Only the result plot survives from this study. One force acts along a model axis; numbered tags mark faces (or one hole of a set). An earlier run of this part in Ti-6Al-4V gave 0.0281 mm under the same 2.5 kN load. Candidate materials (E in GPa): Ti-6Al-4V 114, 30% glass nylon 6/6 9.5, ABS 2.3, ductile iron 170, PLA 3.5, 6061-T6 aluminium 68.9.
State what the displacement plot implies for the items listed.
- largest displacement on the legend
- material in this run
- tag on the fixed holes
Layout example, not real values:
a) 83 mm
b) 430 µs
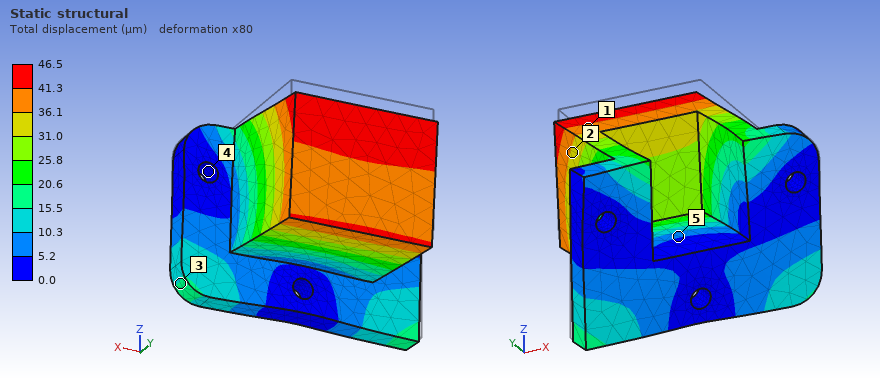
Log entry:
a) 46.5 µm
b) 6061-T6 aluminium
c) 4
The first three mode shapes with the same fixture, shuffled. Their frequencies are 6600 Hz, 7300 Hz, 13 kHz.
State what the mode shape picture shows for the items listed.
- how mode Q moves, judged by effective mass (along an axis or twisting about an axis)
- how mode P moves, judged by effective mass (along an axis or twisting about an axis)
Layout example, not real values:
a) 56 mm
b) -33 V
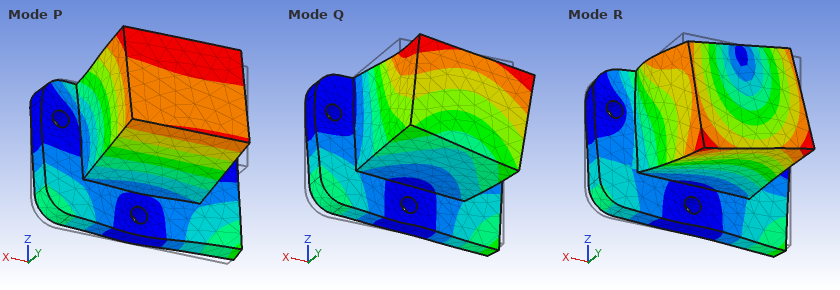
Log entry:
a) along X
b) along Z
